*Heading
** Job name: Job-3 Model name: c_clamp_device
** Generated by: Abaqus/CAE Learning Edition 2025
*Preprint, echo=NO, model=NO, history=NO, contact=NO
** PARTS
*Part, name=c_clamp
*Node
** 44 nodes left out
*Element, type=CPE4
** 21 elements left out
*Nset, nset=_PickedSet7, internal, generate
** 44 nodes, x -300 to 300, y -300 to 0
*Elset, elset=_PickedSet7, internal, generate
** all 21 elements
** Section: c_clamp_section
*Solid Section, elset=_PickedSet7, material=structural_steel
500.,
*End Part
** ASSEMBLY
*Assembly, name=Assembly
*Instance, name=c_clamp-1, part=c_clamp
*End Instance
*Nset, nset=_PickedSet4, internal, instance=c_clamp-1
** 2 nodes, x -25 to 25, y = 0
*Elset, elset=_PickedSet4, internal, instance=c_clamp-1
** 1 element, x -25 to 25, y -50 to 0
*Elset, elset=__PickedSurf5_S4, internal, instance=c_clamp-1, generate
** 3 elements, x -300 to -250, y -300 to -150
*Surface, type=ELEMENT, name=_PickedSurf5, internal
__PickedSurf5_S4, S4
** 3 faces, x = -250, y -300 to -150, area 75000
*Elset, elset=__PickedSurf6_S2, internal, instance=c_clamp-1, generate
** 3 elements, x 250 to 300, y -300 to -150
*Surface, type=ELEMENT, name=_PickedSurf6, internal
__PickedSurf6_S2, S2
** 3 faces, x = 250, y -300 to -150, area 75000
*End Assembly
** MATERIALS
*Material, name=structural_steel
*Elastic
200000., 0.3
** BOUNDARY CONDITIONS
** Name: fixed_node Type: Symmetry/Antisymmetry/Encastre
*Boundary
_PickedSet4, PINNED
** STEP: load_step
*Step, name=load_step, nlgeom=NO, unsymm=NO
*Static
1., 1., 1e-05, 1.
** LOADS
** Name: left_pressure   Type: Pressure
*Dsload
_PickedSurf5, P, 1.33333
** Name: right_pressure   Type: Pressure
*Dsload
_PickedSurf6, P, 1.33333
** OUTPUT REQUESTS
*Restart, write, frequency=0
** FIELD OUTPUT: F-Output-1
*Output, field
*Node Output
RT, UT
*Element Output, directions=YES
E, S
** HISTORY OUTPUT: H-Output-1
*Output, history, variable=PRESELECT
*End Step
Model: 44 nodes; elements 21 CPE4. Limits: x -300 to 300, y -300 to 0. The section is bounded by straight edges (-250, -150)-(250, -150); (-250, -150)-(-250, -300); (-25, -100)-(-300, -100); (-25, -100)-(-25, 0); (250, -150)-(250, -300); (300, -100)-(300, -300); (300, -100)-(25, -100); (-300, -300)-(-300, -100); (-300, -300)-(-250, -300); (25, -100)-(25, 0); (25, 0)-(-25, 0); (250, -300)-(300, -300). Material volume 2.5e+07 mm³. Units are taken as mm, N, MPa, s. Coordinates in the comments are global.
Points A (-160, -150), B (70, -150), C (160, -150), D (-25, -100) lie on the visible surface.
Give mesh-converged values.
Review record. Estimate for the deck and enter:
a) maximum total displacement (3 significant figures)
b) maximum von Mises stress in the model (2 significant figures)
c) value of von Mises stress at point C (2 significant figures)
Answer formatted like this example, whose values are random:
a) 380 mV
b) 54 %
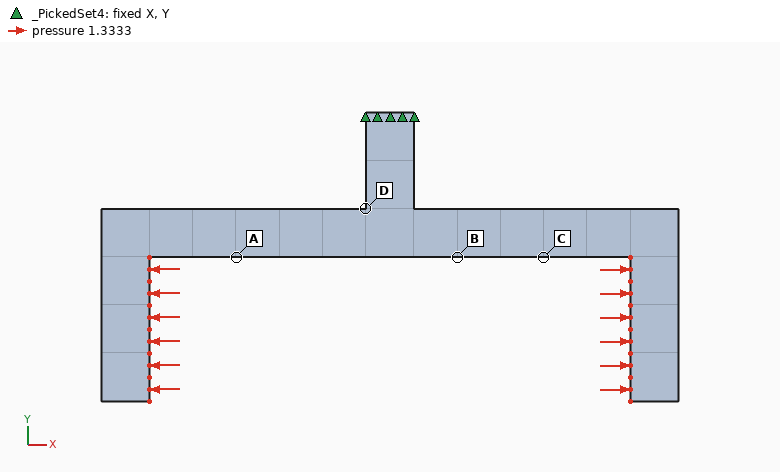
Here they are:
a) 0.595 mm
b) 51 MPa
c) 46 MPa
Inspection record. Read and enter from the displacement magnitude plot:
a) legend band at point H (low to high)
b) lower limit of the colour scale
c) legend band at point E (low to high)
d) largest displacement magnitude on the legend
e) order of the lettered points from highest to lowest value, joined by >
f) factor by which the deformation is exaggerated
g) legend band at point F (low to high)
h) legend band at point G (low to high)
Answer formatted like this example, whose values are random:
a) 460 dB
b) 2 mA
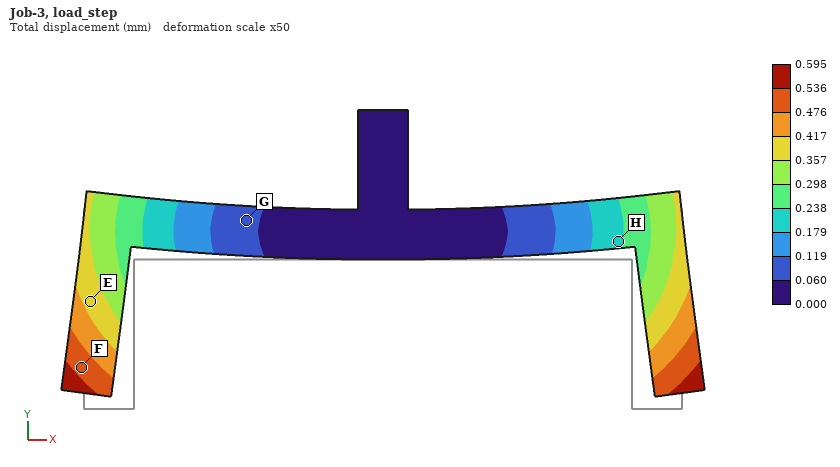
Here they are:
a) 0.179 to 0.238 mm
b) 0.000 mm
c) 0.357 to 0.417 mm
d) 0.595 mm
e) F > E > H > G
f) 50
g) 0.476 to 0.536 mm
h) 0.060 to 0.119 mm
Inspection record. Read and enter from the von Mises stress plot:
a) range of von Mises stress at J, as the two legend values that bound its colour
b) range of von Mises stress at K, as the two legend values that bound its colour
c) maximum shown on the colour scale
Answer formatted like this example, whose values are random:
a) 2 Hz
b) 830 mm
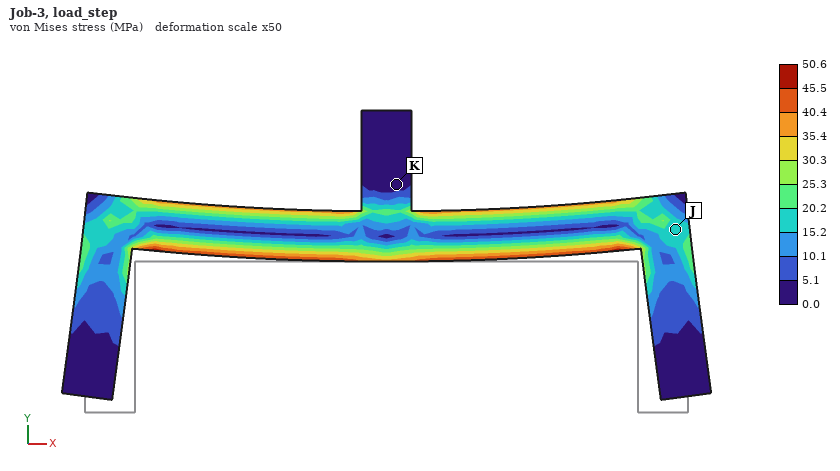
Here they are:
a) 15.2 to 20.2 MPa
b) 0.0 to 5.1 MPa
c) 50.6 MPa
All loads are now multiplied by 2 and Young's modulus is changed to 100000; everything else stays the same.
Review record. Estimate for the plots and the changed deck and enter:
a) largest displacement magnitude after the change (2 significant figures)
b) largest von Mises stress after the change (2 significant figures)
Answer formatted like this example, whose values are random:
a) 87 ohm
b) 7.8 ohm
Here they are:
a) 2.4 mm
b) 100 MPa
